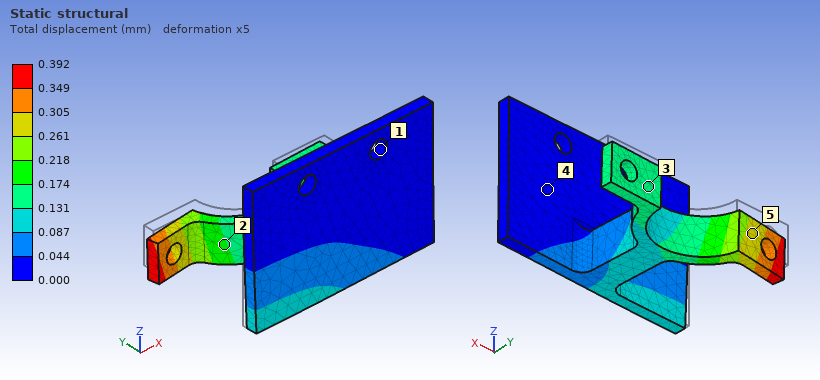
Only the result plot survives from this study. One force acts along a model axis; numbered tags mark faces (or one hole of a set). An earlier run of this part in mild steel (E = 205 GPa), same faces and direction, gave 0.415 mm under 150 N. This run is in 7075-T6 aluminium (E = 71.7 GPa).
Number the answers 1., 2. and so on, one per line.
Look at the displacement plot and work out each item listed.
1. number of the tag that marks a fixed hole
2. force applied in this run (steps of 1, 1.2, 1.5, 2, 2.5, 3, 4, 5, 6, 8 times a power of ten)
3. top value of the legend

1. 1
2. 50 N
3. 0.392 mm
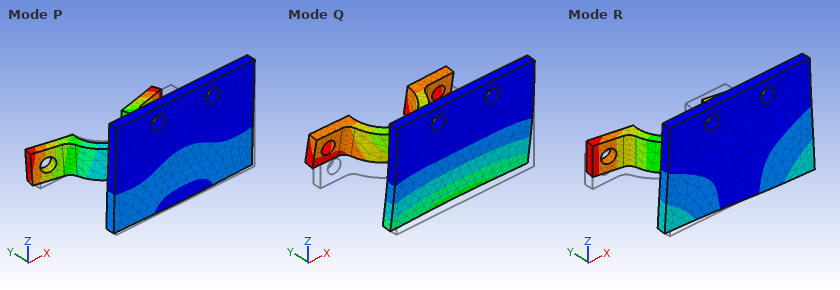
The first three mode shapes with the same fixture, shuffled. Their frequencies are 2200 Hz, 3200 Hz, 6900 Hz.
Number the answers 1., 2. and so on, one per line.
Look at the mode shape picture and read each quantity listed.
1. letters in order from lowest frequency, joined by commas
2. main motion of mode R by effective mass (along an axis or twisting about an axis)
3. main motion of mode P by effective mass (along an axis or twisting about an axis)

1. Q, R, P
2. along X
3. along Y
